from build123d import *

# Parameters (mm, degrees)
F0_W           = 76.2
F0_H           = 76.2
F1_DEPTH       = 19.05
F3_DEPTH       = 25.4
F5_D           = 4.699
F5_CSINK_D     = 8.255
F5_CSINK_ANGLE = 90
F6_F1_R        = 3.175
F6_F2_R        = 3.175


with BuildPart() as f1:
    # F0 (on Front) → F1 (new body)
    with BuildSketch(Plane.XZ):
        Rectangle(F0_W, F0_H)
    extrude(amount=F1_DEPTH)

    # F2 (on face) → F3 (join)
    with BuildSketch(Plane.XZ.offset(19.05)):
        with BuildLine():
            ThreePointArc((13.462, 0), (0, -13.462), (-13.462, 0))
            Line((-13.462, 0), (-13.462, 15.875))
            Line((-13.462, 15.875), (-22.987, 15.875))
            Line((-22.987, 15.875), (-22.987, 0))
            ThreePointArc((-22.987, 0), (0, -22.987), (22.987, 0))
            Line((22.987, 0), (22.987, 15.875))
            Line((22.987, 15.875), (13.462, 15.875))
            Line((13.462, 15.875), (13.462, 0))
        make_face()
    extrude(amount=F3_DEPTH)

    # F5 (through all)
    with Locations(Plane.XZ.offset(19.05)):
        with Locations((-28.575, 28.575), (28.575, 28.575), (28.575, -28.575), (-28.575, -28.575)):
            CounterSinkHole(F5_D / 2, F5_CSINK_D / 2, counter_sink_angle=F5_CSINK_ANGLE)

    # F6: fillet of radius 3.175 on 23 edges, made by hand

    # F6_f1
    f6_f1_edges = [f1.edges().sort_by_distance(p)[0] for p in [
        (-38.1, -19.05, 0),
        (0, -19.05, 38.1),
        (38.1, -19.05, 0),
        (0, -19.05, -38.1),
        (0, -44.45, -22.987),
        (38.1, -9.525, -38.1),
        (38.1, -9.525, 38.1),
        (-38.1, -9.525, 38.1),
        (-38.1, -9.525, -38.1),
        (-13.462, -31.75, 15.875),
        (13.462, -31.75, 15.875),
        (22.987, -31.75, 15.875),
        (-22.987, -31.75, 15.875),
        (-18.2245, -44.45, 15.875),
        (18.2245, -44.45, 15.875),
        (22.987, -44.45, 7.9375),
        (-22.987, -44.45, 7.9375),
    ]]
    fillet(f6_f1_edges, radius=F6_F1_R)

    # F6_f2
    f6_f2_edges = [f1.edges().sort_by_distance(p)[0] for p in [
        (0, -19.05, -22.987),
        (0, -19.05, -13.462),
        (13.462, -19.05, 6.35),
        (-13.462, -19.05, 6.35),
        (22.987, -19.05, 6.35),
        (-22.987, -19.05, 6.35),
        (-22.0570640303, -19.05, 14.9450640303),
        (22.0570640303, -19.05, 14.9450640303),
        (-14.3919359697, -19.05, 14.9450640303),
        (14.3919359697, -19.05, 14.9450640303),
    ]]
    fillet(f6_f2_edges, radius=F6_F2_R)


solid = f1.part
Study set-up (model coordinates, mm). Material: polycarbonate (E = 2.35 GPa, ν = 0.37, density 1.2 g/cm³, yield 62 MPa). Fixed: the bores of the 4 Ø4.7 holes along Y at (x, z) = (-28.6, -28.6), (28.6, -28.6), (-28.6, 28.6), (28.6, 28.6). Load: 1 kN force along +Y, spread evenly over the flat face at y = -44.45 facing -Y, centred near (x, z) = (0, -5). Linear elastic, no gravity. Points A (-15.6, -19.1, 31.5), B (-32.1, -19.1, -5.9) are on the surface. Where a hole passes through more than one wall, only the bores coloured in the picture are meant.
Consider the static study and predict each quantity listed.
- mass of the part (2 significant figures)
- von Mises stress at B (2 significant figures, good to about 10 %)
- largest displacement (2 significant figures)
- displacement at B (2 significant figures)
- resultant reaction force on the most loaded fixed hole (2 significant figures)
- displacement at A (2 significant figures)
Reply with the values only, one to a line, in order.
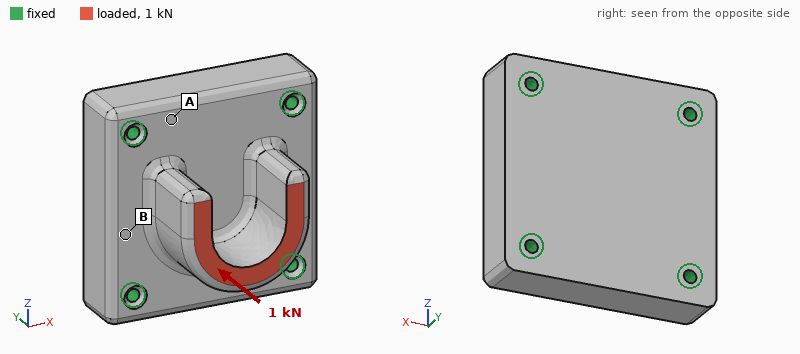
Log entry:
160 g
0.74 MPa
45 µm
16 µm
300 N
7.9 µm
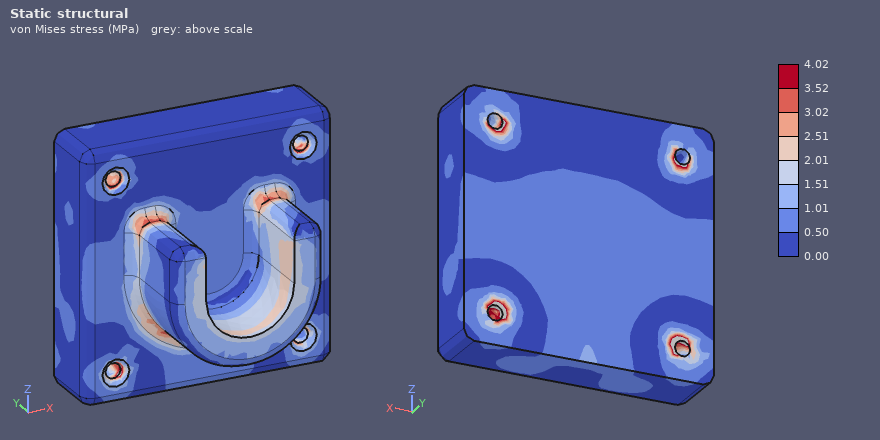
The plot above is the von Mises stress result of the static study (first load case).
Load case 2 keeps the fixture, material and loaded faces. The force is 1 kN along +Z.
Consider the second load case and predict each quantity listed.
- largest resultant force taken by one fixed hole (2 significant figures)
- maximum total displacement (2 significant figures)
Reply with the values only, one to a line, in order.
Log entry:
420 N
0.16 mm
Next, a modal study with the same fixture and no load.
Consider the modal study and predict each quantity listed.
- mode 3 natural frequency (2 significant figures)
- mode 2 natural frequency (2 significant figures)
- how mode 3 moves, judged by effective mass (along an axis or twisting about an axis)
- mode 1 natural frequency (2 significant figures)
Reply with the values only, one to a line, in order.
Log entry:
3800 Hz
3200 Hz
along Z
3200 Hz
